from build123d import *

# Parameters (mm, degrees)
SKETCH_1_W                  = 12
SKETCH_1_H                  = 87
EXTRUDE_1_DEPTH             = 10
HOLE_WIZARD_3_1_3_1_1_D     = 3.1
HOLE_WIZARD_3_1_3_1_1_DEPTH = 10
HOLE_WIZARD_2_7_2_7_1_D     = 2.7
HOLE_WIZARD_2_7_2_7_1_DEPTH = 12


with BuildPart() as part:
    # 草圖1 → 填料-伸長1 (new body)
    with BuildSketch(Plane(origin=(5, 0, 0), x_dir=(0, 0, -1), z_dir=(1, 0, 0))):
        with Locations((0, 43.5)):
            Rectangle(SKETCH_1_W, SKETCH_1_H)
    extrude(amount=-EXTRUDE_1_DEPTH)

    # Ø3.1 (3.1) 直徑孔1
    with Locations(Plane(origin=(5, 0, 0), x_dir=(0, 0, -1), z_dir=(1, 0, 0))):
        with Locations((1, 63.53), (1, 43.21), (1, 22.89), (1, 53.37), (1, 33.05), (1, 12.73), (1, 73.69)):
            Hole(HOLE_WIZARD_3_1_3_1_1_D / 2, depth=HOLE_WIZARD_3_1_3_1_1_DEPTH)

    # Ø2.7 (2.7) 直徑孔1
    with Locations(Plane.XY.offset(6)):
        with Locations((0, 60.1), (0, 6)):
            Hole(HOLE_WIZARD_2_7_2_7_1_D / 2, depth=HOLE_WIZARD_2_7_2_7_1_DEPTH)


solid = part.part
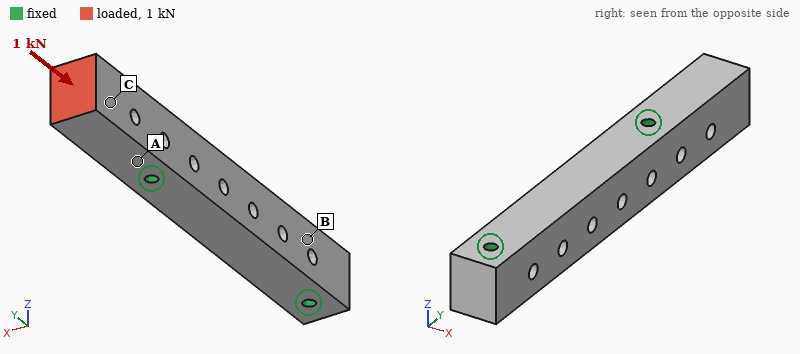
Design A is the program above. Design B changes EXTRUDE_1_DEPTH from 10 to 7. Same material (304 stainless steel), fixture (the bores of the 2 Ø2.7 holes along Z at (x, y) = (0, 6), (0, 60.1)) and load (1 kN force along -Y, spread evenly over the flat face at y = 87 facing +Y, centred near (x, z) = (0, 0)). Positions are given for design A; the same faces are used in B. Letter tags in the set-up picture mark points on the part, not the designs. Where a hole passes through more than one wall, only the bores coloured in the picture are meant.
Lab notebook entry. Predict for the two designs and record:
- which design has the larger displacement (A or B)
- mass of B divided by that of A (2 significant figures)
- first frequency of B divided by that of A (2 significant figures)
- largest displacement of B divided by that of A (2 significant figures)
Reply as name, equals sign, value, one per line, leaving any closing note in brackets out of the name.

which design has the larger displacement = B
mass of B divided by that of A = 0.70
first frequency of B divided by that of A = 0.85
largest displacement of B divided by that of A = 2.3
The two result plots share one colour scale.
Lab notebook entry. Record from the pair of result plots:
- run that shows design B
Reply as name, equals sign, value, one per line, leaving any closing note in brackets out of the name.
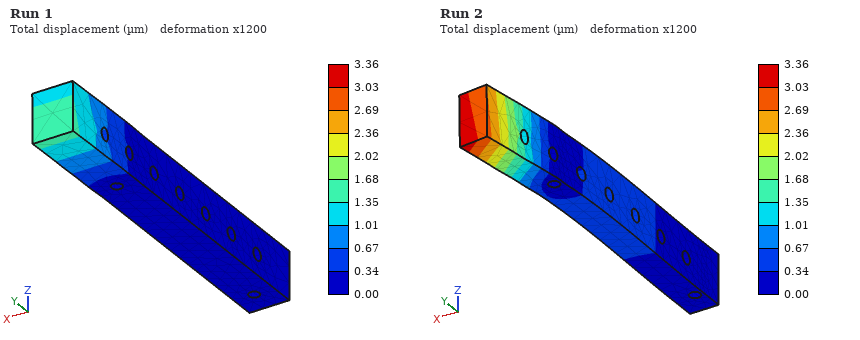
run that shows design B = Run 2
